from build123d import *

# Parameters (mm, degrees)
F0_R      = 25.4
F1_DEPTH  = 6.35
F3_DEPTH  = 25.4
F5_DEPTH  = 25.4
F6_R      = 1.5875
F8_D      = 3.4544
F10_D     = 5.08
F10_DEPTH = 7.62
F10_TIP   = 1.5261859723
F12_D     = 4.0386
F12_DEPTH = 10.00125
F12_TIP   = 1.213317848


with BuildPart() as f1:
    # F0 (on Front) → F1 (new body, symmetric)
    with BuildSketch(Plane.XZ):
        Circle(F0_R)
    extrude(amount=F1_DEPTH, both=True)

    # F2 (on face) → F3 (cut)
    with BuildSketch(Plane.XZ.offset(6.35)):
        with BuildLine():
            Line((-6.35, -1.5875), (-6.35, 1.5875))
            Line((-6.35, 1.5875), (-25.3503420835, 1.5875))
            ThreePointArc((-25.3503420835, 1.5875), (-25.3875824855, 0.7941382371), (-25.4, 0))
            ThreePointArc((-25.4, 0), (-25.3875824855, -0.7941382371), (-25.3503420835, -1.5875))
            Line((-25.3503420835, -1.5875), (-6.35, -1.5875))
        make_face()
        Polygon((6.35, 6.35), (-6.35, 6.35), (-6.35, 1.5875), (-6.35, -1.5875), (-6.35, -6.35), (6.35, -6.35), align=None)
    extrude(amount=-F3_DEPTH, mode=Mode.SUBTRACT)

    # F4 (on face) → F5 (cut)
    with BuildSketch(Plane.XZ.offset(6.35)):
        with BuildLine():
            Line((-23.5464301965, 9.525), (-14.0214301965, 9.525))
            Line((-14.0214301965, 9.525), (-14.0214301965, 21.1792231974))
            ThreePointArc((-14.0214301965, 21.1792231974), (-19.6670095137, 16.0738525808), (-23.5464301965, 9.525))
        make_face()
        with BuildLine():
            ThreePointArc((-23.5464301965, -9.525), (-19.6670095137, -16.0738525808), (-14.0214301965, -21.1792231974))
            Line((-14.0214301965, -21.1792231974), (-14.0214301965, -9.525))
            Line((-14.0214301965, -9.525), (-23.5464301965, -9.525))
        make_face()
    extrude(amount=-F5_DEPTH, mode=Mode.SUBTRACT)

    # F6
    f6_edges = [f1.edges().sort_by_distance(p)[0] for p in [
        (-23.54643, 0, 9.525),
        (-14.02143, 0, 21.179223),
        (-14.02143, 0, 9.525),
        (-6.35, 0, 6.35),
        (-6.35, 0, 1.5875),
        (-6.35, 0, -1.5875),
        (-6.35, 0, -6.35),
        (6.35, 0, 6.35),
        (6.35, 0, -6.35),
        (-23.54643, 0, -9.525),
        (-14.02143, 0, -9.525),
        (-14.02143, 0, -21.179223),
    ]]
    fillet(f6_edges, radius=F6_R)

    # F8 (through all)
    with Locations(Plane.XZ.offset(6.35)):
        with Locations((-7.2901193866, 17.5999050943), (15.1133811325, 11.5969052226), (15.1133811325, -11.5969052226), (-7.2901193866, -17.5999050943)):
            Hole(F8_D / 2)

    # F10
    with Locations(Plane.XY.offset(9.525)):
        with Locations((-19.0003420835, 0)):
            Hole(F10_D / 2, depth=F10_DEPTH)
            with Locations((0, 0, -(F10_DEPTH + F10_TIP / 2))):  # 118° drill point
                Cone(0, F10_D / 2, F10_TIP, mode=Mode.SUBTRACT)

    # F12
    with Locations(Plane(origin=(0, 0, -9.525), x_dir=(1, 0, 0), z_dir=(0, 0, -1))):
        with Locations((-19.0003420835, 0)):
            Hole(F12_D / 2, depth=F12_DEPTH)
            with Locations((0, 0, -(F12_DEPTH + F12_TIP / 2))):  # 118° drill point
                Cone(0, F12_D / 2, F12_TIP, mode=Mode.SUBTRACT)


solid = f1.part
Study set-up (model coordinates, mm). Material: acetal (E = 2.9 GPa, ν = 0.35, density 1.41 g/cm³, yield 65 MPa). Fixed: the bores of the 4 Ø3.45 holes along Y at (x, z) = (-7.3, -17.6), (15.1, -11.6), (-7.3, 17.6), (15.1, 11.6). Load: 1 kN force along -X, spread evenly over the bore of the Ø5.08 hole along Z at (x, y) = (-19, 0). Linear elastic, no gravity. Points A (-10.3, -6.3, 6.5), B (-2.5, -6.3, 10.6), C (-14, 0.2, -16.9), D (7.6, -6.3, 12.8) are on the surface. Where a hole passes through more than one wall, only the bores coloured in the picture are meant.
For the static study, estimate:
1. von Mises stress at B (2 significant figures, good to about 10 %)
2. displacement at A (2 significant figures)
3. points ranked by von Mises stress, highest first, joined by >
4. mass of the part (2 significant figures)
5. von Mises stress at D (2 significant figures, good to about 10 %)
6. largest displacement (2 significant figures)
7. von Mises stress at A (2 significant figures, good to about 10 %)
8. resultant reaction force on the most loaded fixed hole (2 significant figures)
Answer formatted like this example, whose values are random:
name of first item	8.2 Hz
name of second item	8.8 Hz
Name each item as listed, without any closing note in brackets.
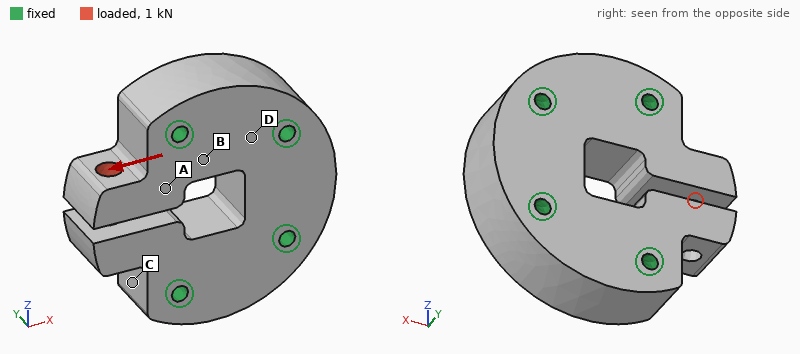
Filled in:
von Mises stress at B	9.0 MPa
displacement at A	0.100 mm
points ranked by von Mises stress, highest first, joined by >	A > B > D > C
mass of the part	29 g
von Mises stress at D	5.8 MPa
largest displacement	0.31 mm
von Mises stress at A	17 MPa
resultant reaction force on the most loaded fixed hole	610 N
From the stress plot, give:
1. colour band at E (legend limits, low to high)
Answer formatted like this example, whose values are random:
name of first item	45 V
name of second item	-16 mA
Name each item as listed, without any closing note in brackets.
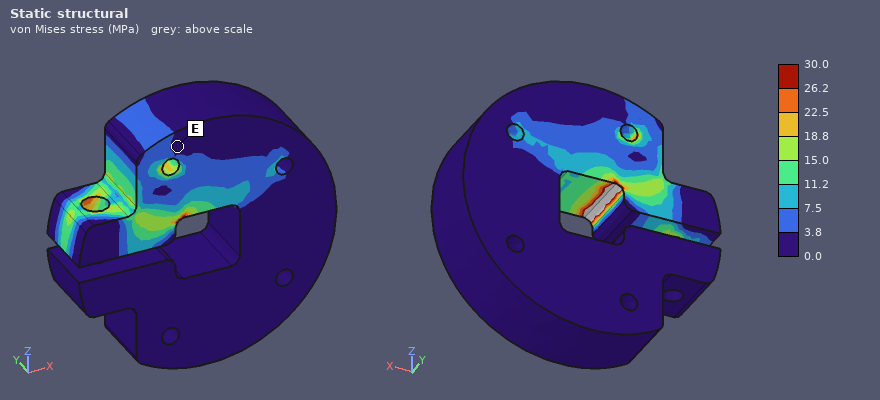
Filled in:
colour band at E	0.0 to 3.8 MPa
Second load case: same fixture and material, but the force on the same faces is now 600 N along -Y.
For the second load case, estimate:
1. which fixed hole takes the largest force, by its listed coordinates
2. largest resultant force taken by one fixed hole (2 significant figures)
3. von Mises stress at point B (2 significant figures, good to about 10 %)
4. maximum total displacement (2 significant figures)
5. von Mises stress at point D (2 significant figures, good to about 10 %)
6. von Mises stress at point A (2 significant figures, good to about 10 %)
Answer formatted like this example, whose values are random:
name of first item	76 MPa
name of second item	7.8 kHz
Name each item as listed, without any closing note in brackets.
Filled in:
which fixed hole takes the largest force, by its listed coordinates	(-7.3, 17.6)
largest resultant force taken by one fixed hole	700 N
von Mises stress at point B	14 MPa
maximum total displacement	0.49 mm
von Mises stress at point D	4.3 MPa
von Mises stress at point A	21 MPa
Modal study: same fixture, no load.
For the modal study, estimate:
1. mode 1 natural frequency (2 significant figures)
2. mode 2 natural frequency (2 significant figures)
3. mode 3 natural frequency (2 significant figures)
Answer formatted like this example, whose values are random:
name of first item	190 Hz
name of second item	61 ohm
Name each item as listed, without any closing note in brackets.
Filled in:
mode 1 natural frequency	5100 Hz
mode 2 natural frequency	5100 Hz
mode 3 natural frequency	5300 Hz
